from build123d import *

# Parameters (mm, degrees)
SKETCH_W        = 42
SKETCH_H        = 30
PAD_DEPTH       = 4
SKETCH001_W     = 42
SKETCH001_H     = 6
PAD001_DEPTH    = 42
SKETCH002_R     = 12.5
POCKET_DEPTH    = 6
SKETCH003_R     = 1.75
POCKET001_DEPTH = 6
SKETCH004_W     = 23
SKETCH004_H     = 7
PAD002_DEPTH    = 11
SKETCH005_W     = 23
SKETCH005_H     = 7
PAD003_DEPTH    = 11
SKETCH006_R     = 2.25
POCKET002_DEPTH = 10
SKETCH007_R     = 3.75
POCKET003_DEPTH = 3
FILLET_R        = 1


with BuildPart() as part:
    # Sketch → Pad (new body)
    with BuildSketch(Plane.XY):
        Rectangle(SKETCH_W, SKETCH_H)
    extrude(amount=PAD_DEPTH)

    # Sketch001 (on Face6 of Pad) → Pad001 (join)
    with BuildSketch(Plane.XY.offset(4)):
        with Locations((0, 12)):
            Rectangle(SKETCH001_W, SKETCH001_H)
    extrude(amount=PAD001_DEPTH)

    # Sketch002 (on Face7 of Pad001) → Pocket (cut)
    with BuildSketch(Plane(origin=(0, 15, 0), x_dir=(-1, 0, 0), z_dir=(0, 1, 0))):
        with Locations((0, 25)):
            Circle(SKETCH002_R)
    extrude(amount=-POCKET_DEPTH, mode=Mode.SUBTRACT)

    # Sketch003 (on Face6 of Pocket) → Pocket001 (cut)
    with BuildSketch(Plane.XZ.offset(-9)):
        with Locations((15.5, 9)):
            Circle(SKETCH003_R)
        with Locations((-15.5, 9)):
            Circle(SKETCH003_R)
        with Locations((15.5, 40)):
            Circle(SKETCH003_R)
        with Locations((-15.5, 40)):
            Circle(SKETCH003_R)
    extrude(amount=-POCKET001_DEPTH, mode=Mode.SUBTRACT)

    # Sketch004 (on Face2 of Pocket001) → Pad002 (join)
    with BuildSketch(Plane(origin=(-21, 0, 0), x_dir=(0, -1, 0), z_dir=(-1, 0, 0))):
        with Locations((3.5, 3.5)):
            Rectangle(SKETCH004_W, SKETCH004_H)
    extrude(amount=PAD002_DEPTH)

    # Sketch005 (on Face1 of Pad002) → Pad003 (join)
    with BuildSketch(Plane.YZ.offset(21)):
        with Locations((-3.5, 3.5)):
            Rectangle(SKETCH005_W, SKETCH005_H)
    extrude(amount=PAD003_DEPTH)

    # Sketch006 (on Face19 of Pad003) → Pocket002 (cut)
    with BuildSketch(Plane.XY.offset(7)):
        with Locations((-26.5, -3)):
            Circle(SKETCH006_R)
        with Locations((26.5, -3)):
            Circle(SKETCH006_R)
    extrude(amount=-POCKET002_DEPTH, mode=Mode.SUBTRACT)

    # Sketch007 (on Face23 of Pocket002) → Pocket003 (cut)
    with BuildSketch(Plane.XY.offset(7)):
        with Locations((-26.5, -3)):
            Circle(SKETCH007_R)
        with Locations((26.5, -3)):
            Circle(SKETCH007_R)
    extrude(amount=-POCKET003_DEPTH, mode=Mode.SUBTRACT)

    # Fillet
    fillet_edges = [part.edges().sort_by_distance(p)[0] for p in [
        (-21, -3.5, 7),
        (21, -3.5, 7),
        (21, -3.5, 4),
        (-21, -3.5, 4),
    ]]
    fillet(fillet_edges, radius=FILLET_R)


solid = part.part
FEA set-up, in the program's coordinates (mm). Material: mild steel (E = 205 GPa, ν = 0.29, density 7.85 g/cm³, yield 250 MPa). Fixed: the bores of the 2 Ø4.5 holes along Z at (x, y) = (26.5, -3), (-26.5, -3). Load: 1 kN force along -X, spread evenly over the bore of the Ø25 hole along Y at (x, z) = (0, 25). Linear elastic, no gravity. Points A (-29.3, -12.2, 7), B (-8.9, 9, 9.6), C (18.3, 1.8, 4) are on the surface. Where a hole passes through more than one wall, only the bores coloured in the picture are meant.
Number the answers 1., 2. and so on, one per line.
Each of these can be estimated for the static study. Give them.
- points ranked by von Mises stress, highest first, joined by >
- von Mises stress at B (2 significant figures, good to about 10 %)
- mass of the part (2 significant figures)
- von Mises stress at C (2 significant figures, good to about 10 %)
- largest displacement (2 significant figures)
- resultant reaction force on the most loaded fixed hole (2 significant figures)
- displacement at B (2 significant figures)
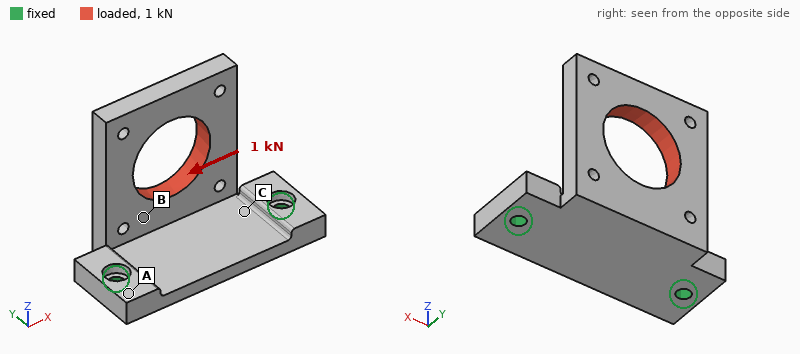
1. C > B > A
2. 25 MPa
3. 120 g
4. 40 MPa
5. 48 µm
6. 780 N
7. 9.9 µm
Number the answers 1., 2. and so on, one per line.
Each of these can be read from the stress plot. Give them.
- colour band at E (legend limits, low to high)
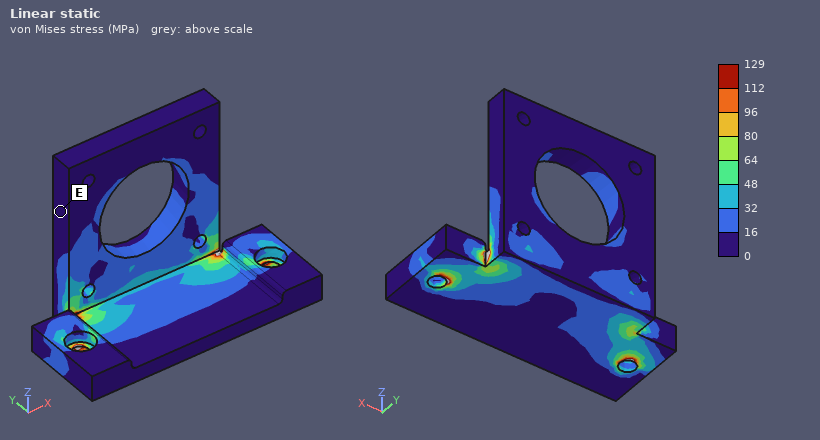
1. 0 to 16 MPa
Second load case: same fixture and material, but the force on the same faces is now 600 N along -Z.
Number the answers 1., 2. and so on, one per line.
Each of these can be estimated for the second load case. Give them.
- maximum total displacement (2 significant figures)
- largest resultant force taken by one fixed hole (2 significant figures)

1. 59 µm
2. 300 N
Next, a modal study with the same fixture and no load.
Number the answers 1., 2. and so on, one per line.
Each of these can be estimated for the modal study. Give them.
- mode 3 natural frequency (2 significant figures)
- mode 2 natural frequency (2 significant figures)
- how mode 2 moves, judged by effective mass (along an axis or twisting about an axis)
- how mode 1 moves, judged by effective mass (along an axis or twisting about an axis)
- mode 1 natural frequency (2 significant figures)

1. 4700 Hz
2. 3300 Hz
3. along X
4. along Y
5. 1200 Hz
